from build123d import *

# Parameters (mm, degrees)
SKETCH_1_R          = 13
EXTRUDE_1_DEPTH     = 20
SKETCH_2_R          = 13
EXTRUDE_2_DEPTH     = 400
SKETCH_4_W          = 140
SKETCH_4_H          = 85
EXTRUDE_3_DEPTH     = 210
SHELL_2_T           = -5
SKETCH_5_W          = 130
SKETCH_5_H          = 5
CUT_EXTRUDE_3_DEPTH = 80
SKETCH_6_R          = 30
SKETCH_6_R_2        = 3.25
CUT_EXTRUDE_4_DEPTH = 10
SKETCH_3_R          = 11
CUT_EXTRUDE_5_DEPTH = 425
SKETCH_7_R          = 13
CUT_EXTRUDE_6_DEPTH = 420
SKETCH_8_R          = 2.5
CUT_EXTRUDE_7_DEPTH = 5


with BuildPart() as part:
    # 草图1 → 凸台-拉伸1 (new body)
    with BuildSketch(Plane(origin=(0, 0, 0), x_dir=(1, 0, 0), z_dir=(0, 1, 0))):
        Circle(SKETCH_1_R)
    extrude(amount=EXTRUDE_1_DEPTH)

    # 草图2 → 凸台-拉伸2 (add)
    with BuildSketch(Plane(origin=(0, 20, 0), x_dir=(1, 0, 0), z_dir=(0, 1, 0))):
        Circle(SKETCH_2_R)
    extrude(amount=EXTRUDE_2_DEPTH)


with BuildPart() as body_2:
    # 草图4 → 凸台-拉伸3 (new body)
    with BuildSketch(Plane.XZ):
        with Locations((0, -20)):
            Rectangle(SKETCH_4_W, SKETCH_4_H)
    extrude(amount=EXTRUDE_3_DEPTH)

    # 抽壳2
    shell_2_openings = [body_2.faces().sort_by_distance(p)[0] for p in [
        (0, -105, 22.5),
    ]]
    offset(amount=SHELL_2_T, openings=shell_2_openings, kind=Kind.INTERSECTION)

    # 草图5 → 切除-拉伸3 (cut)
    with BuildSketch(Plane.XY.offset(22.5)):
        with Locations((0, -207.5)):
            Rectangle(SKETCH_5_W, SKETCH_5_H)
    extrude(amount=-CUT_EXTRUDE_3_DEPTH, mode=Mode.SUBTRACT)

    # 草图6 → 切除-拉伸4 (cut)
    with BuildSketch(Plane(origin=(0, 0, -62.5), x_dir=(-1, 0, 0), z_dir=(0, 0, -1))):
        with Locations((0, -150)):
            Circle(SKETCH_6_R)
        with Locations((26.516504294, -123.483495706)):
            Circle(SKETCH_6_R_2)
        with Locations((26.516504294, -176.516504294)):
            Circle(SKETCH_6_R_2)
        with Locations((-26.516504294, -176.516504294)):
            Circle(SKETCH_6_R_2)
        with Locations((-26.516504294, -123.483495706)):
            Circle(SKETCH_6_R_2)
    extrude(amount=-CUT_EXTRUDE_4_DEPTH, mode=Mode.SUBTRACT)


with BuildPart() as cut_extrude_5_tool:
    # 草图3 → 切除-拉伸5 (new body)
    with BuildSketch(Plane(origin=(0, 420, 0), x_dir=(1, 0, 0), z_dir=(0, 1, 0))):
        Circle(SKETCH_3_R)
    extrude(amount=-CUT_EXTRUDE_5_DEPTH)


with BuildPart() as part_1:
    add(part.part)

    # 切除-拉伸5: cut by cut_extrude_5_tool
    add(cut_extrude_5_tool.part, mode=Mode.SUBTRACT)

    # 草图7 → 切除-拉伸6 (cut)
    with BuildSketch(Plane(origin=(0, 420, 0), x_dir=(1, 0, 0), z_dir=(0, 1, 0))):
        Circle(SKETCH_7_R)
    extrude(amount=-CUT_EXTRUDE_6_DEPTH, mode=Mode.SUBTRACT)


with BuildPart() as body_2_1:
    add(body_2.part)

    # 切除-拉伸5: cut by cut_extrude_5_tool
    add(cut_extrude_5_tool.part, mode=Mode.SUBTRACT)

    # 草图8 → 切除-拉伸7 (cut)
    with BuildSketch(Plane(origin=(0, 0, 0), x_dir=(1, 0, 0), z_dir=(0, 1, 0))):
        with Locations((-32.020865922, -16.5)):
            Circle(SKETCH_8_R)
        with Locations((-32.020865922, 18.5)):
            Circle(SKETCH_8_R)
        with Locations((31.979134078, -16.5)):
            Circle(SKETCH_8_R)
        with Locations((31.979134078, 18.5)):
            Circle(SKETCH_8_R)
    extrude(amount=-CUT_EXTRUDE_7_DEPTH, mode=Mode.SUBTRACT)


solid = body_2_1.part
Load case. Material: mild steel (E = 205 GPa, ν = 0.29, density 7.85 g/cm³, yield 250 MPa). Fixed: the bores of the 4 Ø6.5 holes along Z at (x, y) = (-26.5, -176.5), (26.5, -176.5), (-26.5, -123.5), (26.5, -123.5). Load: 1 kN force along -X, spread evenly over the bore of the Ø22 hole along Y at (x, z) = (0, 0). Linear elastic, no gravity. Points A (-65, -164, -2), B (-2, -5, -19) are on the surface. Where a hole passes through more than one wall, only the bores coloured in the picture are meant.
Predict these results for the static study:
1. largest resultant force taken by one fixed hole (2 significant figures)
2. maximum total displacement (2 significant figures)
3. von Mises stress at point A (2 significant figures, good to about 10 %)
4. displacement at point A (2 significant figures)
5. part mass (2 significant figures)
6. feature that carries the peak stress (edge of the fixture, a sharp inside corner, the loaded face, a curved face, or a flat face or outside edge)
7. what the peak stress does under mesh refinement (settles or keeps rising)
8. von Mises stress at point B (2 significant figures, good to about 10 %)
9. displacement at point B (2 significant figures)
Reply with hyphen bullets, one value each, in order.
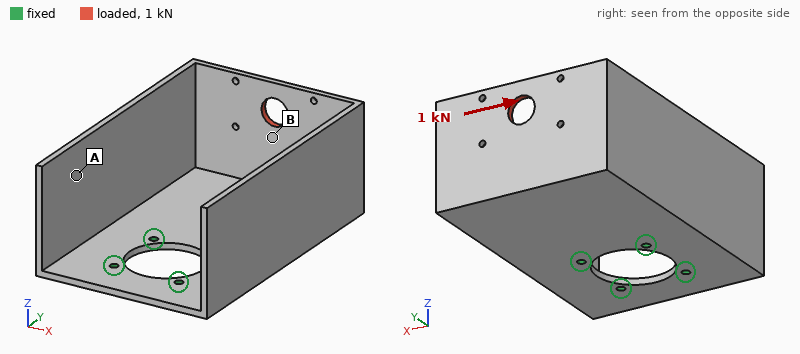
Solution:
- 1.6 kN
- 0.45 mm
- 9.4 MPa
- 0.14 mm
- 2.7 kg
- edge of the fixture
- keeps rising
- 24 MPa
- 0.17 mm
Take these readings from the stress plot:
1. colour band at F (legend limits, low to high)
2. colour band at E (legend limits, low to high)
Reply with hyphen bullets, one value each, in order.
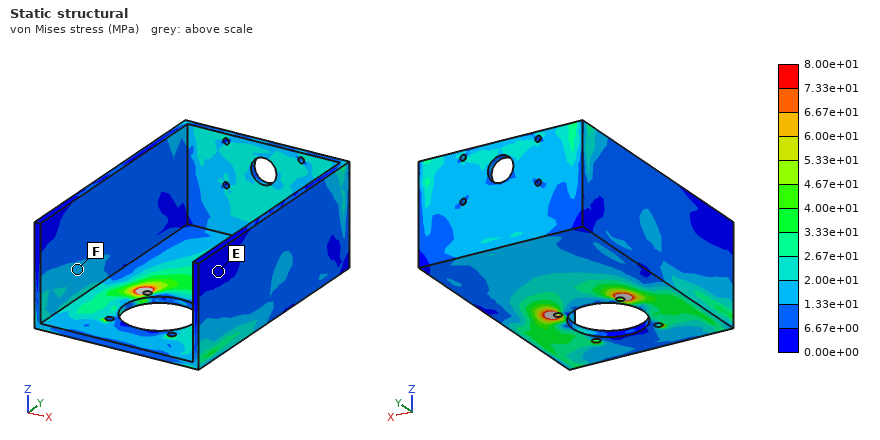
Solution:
- 1.33e+01 to 2.00e+01 MPa
- 0.00e+00 to 6.67e+00 MPa
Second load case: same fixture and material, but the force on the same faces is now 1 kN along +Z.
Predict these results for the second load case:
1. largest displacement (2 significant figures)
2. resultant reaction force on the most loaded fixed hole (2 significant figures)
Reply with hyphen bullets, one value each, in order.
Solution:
- 0.39 mm
- 1.2 kN
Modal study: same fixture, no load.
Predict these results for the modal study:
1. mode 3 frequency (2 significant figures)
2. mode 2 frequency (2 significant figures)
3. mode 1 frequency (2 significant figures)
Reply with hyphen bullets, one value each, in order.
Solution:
- 410 Hz
- 250 Hz
- 250 Hz
